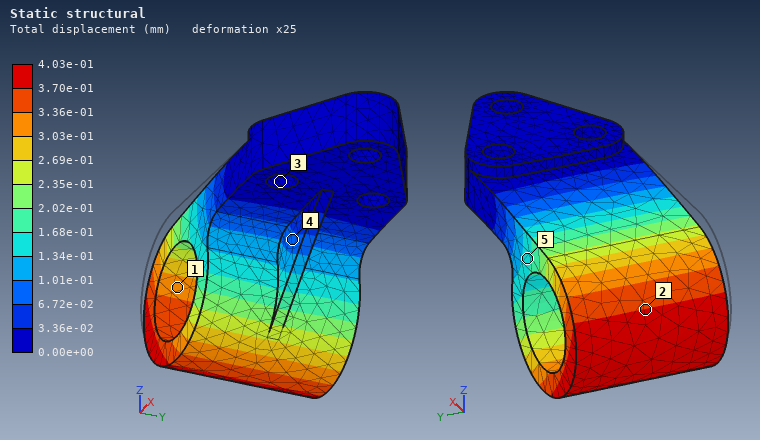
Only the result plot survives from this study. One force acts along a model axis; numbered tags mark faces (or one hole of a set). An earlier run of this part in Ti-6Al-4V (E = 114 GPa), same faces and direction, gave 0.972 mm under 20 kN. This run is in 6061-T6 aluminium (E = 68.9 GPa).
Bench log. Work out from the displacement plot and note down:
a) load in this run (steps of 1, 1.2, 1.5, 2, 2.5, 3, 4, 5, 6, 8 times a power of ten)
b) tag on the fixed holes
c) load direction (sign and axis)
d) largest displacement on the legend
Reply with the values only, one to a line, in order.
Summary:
5 kN
3
-Z
4.03e-01 mm
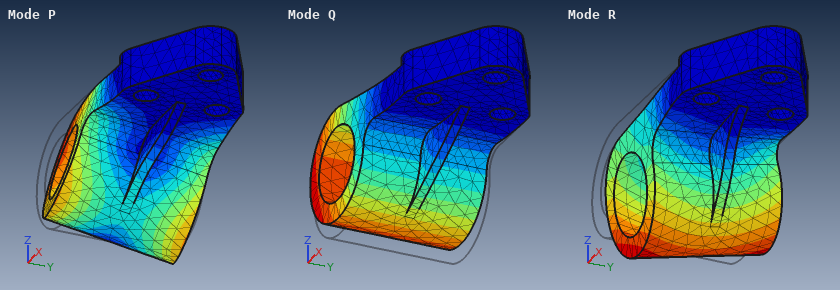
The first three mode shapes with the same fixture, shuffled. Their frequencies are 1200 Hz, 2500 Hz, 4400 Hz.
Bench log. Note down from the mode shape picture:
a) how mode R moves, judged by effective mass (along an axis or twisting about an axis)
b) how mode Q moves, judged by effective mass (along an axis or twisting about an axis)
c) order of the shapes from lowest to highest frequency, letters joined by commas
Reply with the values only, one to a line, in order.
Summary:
along Y
along Z
Q, R, P
